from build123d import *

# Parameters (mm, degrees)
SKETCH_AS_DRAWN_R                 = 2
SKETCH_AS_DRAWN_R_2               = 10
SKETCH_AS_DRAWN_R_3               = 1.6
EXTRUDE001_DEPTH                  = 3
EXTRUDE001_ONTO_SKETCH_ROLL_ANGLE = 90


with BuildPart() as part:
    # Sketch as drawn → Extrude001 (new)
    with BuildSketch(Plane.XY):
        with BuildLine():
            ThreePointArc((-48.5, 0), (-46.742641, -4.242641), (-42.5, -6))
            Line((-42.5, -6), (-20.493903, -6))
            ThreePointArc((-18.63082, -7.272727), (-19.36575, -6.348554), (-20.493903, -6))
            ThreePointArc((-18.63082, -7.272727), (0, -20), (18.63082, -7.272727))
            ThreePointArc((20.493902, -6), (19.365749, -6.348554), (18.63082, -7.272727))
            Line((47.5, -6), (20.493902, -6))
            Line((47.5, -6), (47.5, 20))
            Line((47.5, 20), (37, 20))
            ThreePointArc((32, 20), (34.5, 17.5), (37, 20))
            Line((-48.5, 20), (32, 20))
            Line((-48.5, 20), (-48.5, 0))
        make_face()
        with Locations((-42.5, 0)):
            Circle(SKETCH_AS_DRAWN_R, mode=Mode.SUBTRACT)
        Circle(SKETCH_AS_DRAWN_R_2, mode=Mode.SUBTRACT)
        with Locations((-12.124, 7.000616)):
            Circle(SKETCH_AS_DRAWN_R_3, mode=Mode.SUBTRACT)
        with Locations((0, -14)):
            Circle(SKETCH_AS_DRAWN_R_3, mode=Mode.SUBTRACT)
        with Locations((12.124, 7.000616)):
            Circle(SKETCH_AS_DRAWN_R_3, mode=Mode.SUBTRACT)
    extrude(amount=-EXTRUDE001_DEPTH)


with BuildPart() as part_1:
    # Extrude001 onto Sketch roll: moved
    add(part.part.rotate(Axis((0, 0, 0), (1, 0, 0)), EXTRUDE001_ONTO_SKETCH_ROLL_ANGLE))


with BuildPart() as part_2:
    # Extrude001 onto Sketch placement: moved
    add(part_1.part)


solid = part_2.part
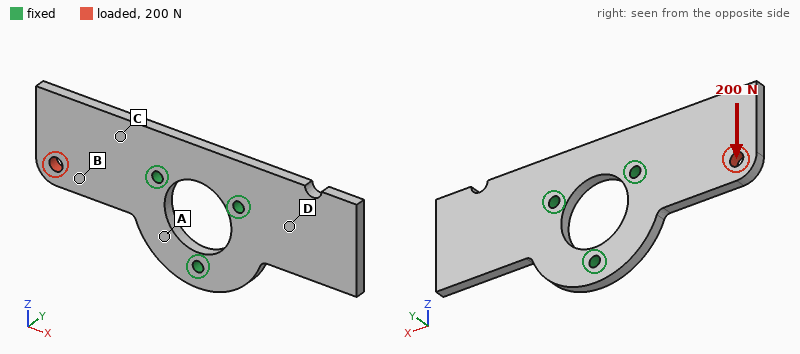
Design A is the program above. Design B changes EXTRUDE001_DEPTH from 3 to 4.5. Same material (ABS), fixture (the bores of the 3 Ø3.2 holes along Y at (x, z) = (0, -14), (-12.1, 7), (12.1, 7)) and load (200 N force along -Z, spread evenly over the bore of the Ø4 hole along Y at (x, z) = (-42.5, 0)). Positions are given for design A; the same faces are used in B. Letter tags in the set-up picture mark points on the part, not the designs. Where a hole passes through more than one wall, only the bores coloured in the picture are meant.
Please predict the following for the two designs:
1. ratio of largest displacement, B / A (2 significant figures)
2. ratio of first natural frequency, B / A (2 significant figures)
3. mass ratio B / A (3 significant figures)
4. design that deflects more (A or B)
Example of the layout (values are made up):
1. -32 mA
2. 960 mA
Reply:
1. 0.67
2. 1.4
3. 1.50
4. A
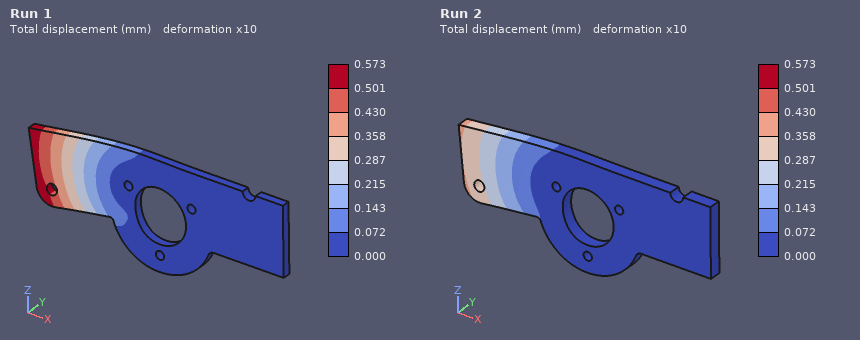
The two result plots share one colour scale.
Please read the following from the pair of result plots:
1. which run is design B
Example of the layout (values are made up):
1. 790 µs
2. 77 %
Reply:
1. Run 2
